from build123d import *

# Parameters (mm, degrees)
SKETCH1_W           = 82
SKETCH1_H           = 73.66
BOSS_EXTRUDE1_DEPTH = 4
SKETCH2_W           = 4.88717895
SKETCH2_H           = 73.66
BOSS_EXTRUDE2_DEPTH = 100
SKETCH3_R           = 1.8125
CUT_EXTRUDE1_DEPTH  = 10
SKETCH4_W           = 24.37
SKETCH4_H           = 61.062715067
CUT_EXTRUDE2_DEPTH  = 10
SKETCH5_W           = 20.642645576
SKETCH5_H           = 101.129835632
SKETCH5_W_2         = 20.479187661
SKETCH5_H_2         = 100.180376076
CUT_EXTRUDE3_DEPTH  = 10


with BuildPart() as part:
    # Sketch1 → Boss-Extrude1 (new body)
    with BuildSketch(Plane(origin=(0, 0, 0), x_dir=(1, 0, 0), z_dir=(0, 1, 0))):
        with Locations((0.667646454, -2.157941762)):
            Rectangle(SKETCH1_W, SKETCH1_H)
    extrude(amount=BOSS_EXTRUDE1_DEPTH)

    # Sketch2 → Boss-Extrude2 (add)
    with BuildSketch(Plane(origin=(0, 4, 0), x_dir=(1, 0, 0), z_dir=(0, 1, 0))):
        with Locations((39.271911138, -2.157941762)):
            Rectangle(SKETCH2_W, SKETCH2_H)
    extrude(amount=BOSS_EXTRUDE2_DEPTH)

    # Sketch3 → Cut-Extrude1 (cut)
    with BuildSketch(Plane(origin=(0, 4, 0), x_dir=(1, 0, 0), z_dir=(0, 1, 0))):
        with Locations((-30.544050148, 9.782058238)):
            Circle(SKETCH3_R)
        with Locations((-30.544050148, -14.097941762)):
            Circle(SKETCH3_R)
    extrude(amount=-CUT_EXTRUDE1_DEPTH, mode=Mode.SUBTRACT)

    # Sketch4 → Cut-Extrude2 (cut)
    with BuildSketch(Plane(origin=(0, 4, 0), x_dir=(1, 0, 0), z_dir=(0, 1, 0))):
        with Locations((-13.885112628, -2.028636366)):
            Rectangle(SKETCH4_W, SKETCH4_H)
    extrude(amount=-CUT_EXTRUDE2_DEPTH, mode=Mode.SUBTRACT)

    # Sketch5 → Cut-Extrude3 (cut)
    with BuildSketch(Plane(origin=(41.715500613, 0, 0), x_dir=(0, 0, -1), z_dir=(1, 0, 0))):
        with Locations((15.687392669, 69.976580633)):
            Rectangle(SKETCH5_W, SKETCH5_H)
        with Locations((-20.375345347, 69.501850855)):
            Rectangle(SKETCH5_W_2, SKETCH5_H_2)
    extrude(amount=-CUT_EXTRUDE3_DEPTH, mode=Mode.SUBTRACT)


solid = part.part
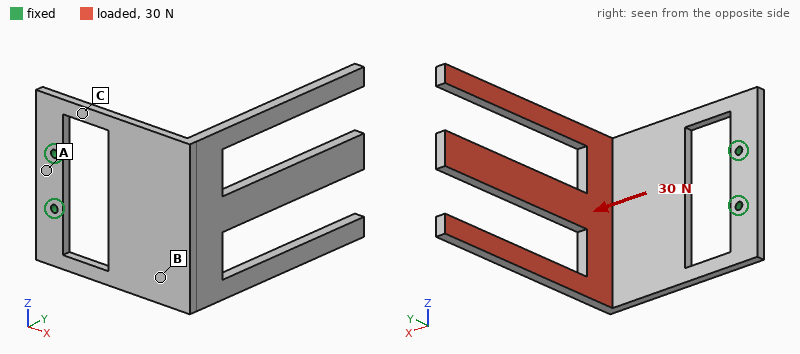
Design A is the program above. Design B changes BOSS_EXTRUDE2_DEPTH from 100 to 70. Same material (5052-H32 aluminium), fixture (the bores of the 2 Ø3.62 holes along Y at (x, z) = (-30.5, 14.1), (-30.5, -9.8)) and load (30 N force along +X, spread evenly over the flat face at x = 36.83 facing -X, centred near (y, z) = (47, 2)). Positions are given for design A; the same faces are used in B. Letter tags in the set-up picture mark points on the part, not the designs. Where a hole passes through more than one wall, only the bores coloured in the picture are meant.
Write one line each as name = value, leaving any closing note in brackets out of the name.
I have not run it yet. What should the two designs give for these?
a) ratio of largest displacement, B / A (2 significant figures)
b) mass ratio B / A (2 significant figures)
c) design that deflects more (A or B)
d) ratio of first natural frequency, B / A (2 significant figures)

ratio of largest displacement, B / A = 0.52
mass ratio B / A = 0.87
design that deflects more = A
ratio of first natural frequency, B / A = 1.3
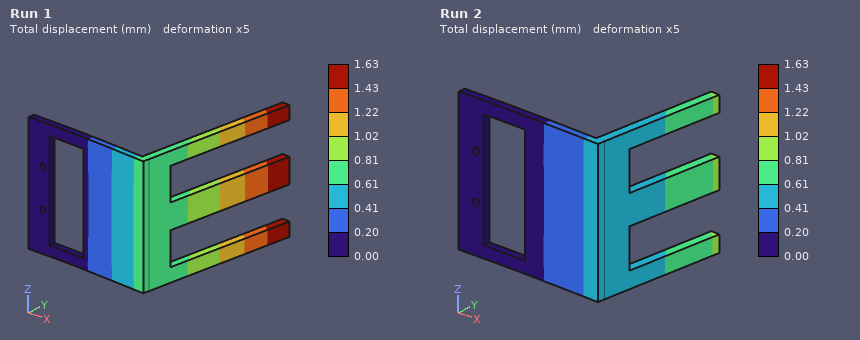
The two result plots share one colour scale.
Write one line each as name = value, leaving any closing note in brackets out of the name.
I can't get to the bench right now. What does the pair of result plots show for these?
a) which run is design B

which run is design B = Run 2
